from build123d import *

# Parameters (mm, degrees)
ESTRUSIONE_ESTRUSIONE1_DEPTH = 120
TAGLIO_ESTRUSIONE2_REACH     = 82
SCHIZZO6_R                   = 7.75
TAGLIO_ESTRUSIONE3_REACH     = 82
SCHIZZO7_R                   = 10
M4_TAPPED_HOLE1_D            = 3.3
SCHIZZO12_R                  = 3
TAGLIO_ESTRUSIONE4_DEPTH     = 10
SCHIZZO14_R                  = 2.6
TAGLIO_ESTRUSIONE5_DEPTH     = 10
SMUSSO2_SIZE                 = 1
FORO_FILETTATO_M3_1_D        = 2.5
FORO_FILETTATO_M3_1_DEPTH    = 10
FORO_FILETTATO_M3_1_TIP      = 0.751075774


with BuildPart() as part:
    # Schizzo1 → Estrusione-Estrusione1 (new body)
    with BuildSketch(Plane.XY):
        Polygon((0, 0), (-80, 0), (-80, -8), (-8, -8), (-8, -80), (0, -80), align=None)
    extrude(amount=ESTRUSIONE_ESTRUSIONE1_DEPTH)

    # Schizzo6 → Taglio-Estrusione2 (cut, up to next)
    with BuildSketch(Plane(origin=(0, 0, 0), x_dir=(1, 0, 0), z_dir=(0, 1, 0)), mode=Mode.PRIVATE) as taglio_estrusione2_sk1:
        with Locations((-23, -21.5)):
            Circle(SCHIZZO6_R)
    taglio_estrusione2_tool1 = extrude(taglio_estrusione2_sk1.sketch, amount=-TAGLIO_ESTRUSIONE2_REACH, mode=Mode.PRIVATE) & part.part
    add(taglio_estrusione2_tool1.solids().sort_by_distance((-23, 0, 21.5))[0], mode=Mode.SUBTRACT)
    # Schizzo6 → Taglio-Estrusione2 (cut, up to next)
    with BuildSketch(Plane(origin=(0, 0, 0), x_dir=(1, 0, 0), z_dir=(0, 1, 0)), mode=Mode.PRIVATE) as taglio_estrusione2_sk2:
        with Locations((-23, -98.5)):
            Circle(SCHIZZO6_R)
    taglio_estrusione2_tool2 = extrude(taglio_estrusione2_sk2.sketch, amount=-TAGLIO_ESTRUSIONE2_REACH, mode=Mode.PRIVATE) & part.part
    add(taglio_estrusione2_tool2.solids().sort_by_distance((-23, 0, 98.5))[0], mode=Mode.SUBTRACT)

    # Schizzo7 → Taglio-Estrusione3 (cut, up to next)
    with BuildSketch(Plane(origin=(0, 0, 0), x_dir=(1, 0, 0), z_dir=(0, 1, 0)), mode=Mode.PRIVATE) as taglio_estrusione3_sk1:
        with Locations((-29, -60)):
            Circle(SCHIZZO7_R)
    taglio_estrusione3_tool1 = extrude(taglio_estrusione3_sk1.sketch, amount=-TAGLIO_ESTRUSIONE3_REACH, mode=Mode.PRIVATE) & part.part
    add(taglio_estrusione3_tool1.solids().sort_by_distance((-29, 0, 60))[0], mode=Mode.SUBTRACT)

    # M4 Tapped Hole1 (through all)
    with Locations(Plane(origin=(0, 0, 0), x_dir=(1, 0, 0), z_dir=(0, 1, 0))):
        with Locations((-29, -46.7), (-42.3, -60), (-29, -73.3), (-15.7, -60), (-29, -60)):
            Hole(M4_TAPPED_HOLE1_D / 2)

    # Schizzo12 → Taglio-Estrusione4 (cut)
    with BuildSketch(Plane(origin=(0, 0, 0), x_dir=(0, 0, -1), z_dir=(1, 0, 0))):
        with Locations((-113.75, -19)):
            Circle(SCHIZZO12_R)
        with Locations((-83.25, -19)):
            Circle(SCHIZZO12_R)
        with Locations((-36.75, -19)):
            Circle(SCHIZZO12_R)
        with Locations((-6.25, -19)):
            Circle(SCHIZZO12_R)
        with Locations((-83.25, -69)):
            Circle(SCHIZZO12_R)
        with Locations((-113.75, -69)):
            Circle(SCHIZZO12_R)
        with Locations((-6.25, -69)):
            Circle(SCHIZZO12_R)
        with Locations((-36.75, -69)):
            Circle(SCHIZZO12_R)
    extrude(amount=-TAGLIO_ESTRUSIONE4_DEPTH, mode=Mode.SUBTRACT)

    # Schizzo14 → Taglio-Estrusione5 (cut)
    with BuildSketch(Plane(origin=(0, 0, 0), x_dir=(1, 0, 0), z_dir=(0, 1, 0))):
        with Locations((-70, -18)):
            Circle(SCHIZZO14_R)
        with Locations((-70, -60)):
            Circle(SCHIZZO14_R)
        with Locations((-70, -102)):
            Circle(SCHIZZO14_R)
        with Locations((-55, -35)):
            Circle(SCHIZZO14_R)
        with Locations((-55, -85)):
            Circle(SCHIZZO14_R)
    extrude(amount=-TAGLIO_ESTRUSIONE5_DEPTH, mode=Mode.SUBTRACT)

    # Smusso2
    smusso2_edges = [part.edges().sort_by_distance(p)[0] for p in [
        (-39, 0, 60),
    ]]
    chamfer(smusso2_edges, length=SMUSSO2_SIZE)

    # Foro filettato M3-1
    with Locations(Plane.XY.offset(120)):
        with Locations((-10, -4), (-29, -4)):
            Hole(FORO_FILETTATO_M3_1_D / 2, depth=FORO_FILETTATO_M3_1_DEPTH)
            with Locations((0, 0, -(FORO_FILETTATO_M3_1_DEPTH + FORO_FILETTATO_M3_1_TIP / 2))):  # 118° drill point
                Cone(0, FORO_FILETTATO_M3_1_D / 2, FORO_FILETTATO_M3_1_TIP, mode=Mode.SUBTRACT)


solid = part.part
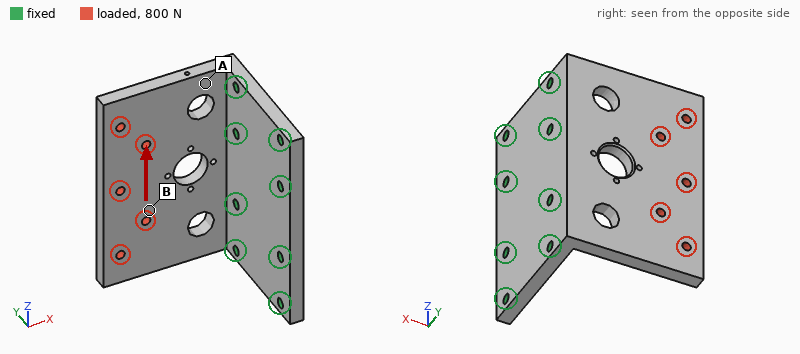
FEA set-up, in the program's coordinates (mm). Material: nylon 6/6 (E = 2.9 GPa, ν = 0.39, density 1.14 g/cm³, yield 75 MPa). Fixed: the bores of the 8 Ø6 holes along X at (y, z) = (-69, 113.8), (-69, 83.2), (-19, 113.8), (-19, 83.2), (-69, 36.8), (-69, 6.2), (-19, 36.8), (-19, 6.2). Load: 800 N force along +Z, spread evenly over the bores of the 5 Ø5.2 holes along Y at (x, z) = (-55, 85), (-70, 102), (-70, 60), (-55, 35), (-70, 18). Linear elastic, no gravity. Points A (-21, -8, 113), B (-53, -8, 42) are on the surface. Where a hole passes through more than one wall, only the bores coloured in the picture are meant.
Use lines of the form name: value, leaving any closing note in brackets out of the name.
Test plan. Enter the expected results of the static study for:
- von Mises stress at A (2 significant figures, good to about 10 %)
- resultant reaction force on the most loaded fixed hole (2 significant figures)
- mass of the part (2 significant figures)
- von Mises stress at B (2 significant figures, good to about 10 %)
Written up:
von Mises stress at A: 6.2 MPa
resultant reaction force on the most loaded fixed hole: 420 N
mass of the part: 160 g
von Mises stress at B: 2.5 MPa
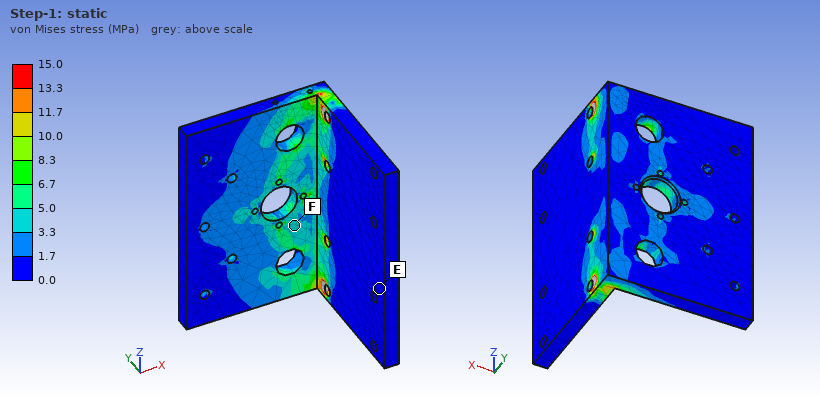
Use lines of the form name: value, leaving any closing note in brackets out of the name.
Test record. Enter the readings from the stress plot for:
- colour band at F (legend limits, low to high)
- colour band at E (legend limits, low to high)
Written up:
colour band at F: 3.3 to 5.0 MPa
colour band at E: 0.0 to 1.7 MPa
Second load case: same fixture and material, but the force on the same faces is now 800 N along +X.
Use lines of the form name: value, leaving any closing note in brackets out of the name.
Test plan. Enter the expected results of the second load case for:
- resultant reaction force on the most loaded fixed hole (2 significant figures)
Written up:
resultant reaction force on the most loaded fixed hole: 250 N
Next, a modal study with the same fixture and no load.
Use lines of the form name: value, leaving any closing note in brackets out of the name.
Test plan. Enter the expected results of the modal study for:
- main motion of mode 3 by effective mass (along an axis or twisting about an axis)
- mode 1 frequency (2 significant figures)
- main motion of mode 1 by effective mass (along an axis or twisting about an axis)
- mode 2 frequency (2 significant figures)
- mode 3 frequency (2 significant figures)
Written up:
main motion of mode 3 by effective mass: along Z
mode 1 frequency: 260 Hz
main motion of mode 1 by effective mass: along Y
mode 2 frequency: 510 Hz
mode 3 frequency: 1300 Hz
